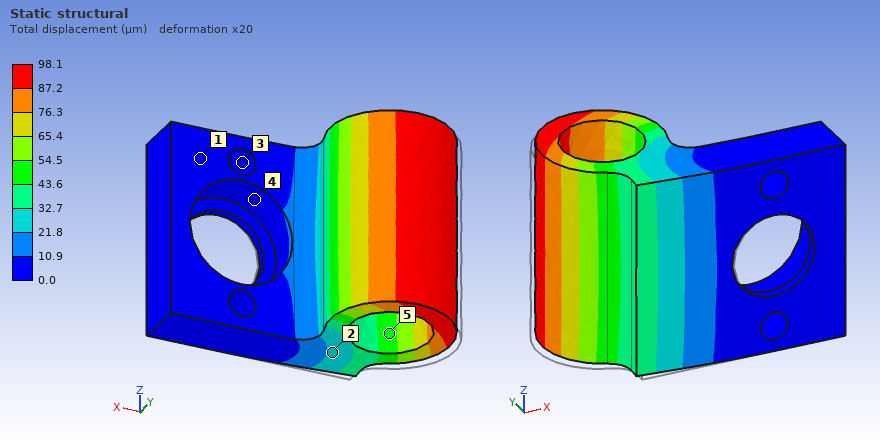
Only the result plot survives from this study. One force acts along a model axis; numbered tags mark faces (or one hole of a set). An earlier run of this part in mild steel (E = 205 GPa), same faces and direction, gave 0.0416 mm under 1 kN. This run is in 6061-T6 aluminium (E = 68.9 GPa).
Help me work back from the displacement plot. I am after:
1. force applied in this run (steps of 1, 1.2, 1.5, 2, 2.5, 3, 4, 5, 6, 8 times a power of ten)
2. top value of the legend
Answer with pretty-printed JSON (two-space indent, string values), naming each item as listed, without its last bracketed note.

{
  "force applied in this run": "800 N",
  "top value of the legend": "98.1 µm"
}
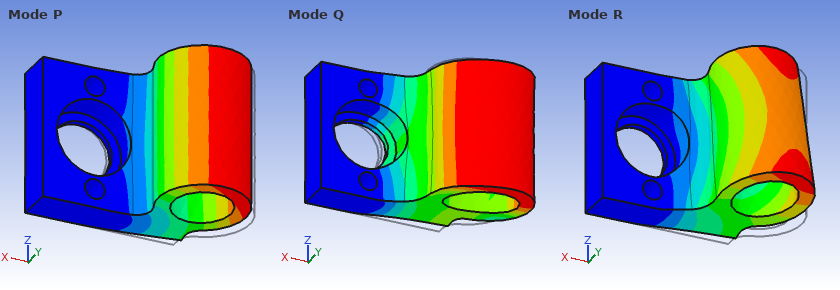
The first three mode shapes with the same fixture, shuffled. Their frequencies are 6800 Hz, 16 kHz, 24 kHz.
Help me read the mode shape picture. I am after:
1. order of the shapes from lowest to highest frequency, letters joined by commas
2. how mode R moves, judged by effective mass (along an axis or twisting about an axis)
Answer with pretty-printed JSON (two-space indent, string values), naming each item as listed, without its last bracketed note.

{
  "order of the shapes from lowest to highest frequency, letters joined by commas": "P, R, Q",
  "how mode R moves, judged by effective mass": "along Z"
}
